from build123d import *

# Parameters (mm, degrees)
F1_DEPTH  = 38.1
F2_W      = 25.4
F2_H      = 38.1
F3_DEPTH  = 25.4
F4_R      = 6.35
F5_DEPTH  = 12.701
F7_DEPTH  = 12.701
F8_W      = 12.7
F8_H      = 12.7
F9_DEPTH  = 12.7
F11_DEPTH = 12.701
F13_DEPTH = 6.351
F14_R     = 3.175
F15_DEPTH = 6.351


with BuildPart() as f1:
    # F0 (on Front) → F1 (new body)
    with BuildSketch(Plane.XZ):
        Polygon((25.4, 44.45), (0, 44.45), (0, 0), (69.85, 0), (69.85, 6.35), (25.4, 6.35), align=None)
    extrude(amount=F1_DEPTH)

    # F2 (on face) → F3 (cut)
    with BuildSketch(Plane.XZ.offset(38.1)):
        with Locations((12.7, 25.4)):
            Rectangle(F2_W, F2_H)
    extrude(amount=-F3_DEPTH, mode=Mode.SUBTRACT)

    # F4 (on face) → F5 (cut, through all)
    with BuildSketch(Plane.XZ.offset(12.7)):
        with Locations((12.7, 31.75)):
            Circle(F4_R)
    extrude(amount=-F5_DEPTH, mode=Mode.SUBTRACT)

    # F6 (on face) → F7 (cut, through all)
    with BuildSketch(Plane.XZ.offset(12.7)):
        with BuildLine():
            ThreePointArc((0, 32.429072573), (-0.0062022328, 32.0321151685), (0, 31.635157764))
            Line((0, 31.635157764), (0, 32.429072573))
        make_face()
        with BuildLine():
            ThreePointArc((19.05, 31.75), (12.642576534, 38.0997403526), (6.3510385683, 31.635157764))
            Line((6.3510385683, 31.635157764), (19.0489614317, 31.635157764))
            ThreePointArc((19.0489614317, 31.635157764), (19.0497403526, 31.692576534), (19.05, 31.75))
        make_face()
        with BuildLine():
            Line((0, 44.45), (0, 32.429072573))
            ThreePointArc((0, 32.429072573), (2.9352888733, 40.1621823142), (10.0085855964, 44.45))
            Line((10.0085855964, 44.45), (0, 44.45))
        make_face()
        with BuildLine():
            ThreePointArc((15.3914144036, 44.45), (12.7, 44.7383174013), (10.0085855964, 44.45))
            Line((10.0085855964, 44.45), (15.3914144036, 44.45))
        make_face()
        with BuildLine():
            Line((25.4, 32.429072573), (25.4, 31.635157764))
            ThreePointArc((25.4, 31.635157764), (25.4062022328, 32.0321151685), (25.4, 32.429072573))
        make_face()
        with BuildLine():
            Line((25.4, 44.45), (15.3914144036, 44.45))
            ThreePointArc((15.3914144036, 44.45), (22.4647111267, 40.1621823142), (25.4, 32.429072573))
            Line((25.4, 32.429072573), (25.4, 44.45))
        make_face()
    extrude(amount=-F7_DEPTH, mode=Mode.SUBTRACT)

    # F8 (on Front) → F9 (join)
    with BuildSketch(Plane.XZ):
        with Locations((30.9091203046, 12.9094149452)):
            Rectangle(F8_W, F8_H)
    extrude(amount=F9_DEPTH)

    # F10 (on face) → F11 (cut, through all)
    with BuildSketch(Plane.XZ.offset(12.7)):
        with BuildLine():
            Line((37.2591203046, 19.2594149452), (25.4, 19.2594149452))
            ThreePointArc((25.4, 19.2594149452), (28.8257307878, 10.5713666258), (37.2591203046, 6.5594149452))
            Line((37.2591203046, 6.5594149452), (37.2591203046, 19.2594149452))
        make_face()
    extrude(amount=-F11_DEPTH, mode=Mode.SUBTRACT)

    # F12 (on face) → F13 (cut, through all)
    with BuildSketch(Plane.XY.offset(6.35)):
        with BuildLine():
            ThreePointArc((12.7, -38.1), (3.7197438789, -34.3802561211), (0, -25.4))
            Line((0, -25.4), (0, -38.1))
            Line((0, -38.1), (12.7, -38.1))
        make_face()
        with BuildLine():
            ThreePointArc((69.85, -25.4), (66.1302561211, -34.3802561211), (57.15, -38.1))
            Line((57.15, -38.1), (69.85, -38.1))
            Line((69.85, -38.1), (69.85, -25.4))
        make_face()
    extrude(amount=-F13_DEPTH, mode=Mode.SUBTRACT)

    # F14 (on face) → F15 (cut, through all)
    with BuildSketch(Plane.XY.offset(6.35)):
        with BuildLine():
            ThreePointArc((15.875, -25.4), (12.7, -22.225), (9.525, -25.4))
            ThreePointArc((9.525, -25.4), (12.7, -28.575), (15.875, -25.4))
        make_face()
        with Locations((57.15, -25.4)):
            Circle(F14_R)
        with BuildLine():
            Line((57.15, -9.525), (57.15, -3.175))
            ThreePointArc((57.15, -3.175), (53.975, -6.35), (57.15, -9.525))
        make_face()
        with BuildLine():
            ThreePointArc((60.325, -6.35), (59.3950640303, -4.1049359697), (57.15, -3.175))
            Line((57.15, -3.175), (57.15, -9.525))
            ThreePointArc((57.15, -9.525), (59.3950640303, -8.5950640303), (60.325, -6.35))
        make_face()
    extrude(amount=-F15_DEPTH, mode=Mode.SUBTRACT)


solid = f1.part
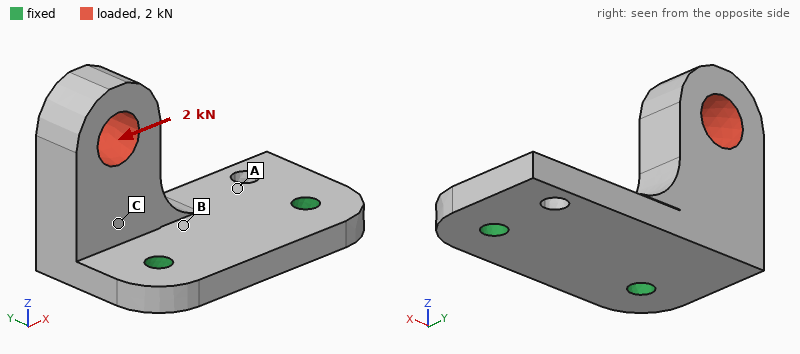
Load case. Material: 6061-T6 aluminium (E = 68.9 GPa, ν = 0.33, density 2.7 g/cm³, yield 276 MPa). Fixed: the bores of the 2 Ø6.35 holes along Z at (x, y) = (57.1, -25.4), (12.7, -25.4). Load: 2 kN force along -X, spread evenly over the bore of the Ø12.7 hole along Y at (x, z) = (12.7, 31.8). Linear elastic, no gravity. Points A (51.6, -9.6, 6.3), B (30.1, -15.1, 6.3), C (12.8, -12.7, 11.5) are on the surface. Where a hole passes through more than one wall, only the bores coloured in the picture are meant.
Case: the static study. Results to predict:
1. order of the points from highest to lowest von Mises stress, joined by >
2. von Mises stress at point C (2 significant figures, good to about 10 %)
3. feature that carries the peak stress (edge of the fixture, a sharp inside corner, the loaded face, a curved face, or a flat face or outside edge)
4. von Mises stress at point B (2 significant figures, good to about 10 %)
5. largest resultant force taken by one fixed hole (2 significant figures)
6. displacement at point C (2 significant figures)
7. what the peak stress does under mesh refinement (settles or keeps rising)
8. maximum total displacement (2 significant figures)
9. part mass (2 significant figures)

B > C > A
41 MPa
a sharp inside corner
74 MPa
1.6 kN
0.061 mm
keeps rising
0.30 mm
71 g
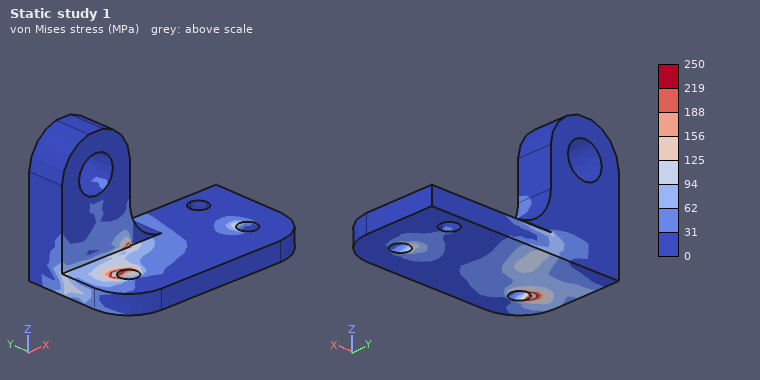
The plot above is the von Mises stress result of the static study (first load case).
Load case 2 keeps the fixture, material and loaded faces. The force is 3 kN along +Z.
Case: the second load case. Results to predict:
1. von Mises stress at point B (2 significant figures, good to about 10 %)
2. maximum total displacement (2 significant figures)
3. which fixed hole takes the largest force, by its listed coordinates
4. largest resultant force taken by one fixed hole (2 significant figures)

67 MPa
0.41 mm
(12.7, -25.4)
2.9 kN
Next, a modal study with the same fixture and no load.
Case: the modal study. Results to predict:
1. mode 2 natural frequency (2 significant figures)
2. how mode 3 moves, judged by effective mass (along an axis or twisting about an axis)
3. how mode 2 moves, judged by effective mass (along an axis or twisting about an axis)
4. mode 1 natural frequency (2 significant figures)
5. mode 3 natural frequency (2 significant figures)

3600 Hz
along Z
along X
2200 Hz
7800 Hz
